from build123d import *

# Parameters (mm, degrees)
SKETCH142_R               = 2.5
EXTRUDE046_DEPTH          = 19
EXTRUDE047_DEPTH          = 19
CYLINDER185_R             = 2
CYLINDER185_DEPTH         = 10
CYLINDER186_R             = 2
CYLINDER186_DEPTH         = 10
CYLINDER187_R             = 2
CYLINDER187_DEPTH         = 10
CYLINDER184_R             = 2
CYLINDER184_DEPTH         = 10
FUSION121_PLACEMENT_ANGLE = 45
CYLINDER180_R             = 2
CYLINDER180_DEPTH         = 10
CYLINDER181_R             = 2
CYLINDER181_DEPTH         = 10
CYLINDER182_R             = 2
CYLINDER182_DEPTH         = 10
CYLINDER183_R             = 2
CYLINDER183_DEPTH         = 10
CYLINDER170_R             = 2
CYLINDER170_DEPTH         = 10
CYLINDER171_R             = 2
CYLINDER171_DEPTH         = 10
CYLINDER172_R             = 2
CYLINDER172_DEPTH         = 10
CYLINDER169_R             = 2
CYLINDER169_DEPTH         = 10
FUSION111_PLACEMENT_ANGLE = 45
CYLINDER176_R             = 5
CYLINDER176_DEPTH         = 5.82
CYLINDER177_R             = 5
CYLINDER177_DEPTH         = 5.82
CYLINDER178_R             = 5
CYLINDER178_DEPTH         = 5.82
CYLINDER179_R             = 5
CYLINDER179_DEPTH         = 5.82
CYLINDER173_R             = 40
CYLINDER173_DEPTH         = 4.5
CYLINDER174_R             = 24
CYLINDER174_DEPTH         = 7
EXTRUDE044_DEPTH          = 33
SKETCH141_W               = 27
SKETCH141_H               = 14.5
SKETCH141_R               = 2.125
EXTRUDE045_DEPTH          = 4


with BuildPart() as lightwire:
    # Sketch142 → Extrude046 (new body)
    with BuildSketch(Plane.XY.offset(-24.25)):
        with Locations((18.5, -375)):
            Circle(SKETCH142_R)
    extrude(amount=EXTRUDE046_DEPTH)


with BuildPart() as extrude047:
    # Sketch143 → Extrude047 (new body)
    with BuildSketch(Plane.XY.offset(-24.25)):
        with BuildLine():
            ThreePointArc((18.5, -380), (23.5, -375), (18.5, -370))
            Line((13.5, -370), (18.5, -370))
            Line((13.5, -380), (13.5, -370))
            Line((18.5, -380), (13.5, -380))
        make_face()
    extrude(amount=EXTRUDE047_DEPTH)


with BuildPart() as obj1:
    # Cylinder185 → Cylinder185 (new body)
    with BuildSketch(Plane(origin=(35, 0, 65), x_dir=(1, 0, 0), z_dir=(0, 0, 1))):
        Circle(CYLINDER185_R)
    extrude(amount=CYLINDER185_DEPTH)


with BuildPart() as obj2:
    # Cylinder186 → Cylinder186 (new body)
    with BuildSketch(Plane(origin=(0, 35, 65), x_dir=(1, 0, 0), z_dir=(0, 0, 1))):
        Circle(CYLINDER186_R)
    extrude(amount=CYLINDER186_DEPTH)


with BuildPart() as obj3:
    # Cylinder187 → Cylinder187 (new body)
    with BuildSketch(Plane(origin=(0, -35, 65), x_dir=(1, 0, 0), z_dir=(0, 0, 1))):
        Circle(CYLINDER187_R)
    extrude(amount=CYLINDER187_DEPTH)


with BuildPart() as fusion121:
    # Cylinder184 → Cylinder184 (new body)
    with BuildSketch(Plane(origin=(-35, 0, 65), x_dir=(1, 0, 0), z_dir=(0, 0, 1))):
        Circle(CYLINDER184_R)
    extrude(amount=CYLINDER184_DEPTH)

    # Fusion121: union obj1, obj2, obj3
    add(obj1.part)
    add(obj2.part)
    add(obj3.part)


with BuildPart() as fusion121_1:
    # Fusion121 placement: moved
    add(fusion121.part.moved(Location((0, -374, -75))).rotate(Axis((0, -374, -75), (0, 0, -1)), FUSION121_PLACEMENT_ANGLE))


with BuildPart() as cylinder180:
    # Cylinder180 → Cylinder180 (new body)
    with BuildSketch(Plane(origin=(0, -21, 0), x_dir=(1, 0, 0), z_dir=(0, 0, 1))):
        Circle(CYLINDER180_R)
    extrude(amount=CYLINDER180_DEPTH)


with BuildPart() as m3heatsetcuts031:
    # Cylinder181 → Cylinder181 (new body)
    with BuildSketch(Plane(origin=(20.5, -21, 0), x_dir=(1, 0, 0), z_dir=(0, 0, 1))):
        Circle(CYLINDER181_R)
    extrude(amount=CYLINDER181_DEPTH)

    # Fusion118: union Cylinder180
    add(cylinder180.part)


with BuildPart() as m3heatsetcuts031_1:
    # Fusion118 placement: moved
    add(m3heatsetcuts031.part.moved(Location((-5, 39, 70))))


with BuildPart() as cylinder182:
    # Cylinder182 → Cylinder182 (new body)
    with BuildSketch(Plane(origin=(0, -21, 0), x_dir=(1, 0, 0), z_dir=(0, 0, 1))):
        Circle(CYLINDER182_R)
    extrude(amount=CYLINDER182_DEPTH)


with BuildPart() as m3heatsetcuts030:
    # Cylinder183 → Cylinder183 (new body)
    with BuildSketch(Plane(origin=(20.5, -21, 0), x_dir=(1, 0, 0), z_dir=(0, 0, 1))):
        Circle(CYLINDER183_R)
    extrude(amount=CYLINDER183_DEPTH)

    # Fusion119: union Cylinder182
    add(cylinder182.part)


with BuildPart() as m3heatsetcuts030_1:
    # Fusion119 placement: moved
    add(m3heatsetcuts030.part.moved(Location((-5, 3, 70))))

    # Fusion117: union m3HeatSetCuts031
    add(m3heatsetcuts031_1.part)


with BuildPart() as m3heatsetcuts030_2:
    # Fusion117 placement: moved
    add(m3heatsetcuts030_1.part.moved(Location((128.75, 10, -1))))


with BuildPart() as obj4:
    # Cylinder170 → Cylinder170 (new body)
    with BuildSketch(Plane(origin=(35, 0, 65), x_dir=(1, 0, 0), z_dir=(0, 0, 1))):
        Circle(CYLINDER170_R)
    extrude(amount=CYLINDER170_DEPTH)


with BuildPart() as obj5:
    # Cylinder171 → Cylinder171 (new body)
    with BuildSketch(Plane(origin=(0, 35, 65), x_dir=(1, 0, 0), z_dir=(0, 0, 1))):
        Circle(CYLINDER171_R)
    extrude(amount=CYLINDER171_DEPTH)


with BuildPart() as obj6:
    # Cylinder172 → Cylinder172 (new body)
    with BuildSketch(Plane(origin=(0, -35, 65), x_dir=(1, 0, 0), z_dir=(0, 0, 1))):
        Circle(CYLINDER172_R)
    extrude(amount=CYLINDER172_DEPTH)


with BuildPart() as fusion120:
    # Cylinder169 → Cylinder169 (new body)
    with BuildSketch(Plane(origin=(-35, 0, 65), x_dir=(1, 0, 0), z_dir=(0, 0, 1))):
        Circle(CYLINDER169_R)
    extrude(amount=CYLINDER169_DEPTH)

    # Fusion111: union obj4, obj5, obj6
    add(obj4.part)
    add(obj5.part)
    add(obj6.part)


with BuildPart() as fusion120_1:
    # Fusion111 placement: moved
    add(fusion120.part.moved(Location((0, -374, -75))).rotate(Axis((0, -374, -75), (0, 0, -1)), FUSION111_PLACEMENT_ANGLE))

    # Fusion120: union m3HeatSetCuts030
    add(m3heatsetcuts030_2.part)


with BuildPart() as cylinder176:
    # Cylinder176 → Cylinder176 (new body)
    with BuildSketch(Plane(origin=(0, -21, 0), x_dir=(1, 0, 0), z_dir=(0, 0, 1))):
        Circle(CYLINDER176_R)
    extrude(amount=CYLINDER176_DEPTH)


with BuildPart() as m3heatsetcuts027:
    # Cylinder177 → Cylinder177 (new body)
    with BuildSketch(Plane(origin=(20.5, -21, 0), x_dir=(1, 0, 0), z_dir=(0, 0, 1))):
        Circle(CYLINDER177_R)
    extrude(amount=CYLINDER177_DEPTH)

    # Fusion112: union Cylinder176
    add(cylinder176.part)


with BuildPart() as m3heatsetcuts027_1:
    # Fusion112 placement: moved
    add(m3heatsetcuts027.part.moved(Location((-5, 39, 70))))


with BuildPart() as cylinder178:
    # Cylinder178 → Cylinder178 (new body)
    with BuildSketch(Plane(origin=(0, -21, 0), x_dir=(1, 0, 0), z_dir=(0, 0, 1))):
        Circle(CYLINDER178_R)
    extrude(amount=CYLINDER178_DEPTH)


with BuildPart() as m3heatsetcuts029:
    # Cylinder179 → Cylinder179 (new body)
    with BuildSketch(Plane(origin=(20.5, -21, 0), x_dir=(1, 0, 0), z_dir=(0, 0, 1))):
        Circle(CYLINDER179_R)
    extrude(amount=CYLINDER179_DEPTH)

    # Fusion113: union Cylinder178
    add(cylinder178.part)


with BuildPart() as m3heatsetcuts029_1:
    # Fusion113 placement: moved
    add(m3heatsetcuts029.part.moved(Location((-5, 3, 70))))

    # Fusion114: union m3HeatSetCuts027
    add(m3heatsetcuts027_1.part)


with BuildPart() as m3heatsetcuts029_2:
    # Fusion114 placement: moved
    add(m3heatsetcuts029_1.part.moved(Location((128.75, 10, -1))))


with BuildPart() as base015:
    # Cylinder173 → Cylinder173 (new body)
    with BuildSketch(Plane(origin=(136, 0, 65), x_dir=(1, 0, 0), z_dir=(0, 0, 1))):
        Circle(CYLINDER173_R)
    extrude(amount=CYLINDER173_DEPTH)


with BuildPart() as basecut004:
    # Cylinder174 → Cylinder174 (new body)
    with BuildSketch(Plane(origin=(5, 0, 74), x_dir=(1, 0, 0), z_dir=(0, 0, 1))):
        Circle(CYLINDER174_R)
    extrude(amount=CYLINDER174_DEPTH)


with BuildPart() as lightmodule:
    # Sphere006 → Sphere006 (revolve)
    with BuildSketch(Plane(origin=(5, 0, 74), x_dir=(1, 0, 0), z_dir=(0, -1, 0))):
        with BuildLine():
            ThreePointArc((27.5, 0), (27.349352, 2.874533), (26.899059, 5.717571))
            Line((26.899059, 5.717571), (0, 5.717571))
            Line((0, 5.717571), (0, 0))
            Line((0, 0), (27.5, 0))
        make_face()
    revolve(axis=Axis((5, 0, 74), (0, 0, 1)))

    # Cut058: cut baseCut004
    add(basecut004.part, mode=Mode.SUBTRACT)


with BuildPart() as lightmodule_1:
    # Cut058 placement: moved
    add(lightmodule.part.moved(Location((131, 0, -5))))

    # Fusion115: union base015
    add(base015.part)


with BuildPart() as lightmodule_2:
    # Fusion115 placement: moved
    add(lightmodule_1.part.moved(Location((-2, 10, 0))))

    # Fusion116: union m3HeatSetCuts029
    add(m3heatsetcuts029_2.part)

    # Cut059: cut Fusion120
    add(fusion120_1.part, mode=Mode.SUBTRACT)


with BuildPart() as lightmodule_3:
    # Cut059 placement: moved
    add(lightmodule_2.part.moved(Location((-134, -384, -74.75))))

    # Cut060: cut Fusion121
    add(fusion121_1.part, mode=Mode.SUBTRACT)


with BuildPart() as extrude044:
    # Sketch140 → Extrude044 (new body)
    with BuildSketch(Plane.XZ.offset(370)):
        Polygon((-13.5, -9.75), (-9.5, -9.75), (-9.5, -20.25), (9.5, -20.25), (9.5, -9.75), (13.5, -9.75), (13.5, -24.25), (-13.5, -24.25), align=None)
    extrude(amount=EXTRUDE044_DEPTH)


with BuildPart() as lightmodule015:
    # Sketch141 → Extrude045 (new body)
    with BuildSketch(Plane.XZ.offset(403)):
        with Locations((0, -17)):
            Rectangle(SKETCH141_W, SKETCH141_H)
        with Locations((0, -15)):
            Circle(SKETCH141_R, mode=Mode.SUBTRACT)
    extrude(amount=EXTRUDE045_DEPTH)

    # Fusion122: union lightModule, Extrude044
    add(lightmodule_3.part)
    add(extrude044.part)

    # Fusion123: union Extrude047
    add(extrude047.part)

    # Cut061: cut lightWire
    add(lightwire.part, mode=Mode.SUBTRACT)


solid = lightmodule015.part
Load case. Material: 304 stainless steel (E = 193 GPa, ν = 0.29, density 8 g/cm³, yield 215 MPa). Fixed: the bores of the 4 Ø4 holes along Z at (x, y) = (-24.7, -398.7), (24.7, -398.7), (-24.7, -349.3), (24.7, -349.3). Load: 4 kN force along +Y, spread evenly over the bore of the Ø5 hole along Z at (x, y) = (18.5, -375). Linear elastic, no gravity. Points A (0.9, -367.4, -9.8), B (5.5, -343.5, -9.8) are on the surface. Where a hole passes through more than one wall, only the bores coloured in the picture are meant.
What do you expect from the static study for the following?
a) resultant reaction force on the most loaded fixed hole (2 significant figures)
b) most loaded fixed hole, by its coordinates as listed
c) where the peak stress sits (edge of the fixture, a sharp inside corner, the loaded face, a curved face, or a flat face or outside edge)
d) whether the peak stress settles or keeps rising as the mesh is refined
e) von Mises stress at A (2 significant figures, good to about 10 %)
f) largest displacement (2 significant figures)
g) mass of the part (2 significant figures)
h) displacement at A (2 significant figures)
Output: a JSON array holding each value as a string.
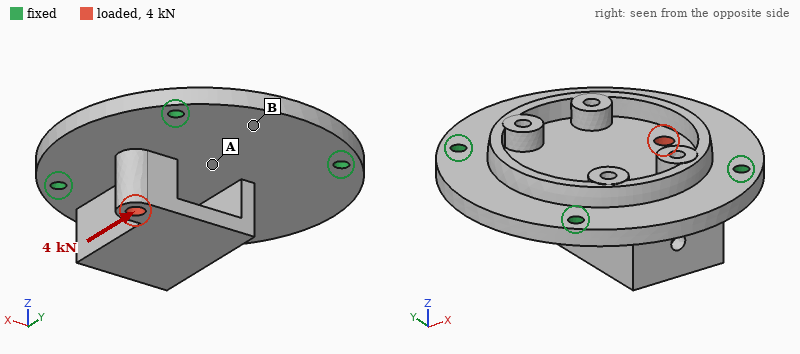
["1.8 kN", "(24.7, -398.7)", "edge of the fixture", "keeps rising", "20 MPa", "21 µm", "280 g", "7.0 µm"]
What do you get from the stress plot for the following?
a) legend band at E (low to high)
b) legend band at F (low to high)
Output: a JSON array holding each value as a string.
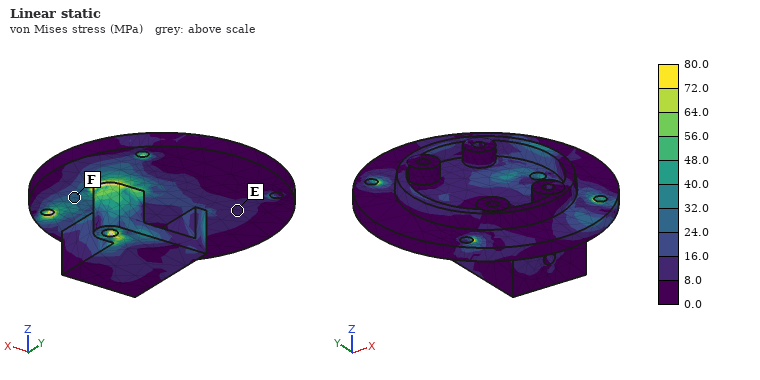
["8.0 to 16.0 MPa", "24.0 to 32.0 MPa"]
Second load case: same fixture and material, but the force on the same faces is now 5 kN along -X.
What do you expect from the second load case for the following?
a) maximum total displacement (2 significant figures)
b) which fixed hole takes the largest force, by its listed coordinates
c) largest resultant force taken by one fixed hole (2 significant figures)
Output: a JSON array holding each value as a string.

["20 µm", "(24.7, -398.7)", "1.7 kN"]
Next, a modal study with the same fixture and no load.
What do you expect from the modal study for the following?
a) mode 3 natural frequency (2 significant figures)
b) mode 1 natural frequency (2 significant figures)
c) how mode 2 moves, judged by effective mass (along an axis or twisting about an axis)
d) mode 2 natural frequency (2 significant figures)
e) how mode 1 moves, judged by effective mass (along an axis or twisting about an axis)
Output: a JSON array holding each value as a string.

["8300 Hz", "6100 Hz", "along Z", "7600 Hz", "along Z"]
